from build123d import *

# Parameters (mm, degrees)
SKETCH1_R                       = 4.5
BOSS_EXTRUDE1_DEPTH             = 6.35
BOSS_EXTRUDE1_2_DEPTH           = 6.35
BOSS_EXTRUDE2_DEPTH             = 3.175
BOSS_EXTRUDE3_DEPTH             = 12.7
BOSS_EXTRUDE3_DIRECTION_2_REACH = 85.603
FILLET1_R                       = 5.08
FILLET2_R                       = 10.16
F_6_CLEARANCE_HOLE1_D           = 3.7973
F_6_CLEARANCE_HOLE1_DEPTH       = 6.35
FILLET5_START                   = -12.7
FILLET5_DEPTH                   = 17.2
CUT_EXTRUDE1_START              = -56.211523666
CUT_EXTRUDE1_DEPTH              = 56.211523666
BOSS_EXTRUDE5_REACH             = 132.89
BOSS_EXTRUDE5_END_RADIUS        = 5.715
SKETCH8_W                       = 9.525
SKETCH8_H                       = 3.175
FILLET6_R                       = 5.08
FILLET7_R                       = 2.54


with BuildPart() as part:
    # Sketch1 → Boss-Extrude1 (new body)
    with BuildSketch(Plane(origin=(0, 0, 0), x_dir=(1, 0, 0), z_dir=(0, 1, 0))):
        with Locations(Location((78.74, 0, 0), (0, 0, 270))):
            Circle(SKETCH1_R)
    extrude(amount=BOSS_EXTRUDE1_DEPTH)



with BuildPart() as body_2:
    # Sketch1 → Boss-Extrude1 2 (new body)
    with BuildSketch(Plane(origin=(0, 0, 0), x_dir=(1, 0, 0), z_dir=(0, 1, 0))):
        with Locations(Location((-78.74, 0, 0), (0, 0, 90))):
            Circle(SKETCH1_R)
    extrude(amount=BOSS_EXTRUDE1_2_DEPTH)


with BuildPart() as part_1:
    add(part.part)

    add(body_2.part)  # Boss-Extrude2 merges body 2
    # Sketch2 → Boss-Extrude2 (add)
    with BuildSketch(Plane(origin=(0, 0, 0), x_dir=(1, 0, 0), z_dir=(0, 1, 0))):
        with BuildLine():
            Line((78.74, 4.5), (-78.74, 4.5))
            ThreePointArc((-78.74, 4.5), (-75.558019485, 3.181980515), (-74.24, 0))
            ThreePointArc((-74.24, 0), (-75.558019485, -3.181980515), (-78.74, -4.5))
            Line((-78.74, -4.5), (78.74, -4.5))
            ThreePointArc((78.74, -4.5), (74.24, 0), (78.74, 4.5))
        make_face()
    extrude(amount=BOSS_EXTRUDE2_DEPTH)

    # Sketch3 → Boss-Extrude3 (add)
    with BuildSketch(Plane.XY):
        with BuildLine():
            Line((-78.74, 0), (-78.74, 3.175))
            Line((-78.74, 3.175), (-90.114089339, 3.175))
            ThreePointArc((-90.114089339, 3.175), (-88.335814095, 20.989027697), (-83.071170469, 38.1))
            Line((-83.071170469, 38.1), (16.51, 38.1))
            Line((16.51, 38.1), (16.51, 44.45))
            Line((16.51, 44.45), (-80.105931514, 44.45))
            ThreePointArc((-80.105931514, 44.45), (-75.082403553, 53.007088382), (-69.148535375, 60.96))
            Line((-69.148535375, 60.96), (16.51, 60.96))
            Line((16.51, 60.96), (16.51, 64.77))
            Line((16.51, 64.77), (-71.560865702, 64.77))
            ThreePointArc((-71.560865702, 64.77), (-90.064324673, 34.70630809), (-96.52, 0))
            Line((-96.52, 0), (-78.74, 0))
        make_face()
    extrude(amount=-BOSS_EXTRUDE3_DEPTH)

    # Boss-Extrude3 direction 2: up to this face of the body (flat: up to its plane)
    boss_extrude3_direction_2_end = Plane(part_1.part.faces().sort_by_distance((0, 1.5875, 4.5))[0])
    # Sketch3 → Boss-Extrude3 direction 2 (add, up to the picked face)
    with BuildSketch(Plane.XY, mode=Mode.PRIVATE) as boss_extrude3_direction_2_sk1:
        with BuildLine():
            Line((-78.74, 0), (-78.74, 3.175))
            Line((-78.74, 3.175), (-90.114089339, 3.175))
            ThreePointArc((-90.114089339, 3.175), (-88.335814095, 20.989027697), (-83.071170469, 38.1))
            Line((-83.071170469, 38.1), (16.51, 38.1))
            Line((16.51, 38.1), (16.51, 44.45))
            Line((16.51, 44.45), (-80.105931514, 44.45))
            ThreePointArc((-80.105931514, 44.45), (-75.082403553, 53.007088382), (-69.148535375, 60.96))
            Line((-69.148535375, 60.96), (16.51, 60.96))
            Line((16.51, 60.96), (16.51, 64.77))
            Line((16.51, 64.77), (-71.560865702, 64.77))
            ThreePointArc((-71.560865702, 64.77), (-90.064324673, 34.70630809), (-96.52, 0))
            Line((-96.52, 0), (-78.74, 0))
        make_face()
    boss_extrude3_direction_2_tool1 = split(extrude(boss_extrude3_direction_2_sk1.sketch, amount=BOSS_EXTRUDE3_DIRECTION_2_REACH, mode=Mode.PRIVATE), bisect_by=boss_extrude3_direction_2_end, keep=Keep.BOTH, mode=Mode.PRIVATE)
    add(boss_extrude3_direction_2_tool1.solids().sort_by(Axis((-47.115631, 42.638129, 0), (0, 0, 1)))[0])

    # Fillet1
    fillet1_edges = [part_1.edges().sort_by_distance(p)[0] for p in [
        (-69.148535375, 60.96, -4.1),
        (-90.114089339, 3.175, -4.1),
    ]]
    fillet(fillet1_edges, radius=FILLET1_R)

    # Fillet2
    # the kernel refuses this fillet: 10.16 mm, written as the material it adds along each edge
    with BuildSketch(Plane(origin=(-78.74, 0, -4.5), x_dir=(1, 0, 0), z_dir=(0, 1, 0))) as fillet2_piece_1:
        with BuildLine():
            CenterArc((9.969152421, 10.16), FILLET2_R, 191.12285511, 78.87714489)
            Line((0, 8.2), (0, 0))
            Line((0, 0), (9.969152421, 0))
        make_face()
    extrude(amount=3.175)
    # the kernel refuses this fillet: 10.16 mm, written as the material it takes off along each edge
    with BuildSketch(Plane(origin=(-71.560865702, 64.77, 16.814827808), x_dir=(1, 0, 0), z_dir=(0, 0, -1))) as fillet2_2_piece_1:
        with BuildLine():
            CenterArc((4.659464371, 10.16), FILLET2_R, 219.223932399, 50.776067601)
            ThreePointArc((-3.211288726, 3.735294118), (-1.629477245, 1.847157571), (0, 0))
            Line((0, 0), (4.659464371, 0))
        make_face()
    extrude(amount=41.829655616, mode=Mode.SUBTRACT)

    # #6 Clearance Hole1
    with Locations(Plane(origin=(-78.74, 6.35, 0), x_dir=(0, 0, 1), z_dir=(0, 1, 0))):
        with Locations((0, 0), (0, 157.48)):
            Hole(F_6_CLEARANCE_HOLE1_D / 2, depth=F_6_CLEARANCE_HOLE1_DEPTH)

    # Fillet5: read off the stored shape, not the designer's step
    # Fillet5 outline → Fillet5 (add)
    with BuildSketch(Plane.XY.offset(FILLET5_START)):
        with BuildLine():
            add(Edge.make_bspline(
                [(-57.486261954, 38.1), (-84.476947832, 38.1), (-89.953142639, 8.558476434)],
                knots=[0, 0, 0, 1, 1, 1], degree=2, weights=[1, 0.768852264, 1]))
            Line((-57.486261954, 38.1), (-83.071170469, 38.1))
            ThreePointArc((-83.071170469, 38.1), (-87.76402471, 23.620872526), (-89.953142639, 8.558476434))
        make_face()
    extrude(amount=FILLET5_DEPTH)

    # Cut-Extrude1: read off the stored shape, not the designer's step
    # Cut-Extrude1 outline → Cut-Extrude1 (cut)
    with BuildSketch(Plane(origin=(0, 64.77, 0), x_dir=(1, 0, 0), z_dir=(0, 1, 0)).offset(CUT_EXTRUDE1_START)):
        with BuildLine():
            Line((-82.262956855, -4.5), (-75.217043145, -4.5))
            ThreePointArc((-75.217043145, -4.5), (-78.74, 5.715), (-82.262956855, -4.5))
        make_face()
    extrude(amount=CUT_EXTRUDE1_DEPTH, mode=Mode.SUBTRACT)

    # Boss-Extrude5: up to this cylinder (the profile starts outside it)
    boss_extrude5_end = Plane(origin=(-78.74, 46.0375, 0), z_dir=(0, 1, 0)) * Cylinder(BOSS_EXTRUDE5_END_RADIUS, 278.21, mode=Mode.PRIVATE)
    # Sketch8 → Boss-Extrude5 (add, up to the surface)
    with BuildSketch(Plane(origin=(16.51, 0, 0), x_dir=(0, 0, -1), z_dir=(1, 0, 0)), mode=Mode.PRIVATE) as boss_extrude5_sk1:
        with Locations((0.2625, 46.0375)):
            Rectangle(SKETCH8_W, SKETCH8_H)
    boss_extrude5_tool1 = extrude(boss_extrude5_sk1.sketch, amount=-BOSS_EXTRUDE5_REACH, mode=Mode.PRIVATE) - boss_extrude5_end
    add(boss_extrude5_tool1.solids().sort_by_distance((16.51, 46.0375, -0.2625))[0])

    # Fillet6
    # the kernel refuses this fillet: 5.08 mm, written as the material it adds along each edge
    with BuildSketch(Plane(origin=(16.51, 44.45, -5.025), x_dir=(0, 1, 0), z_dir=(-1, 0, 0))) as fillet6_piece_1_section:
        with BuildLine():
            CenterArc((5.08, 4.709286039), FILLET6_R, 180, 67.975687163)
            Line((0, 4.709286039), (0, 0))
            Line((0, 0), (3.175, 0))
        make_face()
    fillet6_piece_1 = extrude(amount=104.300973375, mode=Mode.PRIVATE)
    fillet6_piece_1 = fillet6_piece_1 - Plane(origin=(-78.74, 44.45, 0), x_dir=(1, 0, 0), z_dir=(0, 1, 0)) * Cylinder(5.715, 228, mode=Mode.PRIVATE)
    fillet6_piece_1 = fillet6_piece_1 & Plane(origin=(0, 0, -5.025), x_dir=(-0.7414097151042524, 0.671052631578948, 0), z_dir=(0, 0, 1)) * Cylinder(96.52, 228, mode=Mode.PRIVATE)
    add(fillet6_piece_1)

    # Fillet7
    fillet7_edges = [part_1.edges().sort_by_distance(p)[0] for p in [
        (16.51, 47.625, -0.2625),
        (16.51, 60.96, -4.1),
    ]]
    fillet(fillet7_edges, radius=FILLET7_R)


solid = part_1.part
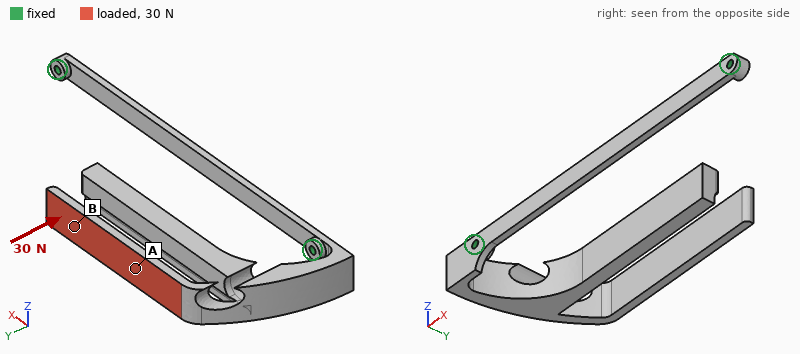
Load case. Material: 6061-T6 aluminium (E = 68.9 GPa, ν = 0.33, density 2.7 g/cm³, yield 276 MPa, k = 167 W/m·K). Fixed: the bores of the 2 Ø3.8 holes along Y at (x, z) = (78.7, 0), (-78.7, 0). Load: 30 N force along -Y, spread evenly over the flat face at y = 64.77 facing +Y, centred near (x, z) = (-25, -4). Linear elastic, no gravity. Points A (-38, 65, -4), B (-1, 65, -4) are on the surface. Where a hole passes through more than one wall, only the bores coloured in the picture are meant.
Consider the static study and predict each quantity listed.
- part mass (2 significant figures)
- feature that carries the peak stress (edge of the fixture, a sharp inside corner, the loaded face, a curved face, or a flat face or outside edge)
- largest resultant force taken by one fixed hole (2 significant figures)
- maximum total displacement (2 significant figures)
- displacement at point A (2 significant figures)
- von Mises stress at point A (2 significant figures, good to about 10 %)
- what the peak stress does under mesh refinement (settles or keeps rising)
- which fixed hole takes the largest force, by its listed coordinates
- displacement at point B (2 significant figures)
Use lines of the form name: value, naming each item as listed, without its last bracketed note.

part mass: 87 g
feature that carries the peak stress: a sharp inside corner
largest resultant force taken by one fixed hole: 30 N
maximum total displacement: 1.9 mm
displacement at point A: 0.85 mm
von Mises stress at point A: 13 MPa
what the peak stress does under mesh refinement: keeps rising
which fixed hole takes the largest force, by its listed coordinates: (-78.7, 0)
displacement at point B: 1.6 mm
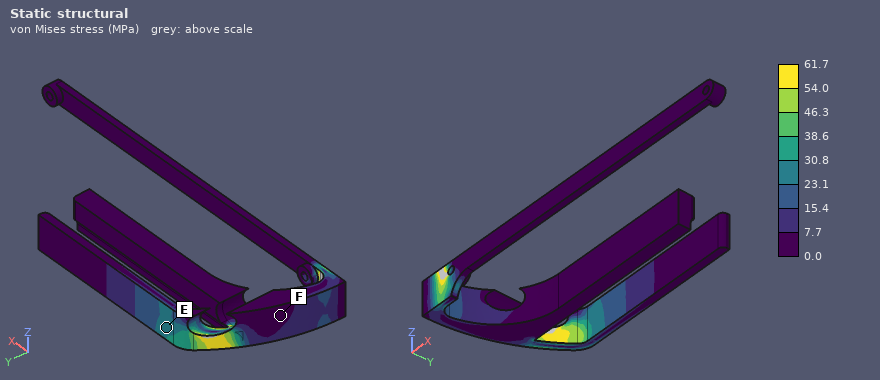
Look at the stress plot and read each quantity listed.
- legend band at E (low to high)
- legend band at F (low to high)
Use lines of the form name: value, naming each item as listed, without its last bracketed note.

legend band at E: 23.1 to 30.8 MPa
legend band at F: 0.0 to 7.7 MPa
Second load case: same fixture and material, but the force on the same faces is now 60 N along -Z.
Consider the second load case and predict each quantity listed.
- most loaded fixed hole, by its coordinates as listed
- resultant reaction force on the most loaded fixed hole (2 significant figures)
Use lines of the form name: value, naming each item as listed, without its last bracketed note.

most loaded fixed hole, by its coordinates as listed: (-78.7, 0)
resultant reaction force on the most loaded fixed hole: 59 N
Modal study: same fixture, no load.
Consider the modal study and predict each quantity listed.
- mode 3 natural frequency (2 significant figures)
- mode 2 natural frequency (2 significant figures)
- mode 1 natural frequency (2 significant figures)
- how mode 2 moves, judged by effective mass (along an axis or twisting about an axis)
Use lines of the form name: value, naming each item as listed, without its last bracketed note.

mode 3 natural frequency: 300 Hz
mode 2 natural frequency: 220 Hz
mode 1 natural frequency: 140 Hz
how mode 2 moves, judged by effective mass: along Z
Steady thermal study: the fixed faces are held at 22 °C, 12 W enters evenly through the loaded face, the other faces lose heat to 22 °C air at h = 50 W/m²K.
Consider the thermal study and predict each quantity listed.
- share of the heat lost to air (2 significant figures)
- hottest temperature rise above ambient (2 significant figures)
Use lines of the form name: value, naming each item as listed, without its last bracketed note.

share of the heat lost to air: 76 %
hottest temperature rise above ambient: 58 K
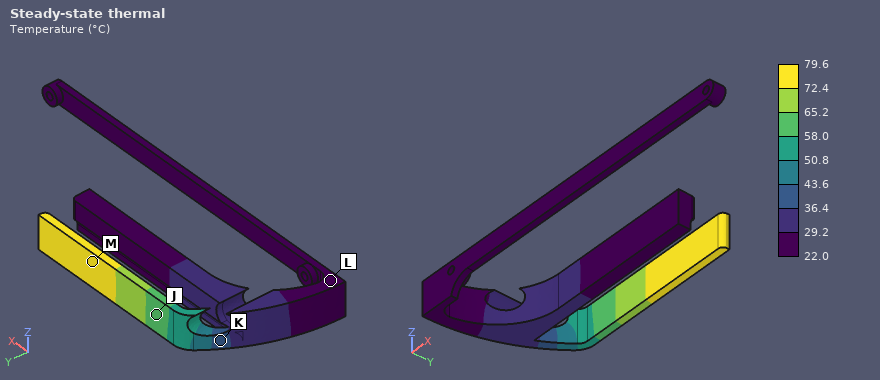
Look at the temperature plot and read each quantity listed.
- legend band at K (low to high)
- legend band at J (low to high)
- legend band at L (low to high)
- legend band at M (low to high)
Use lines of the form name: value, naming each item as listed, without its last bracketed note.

legend band at K: 36.4 to 43.6 °C
legend band at J: 58.0 to 65.2 °C
legend band at L: 22.0 to 29.2 °C
legend band at M: 72.4 to 79.6 °C
